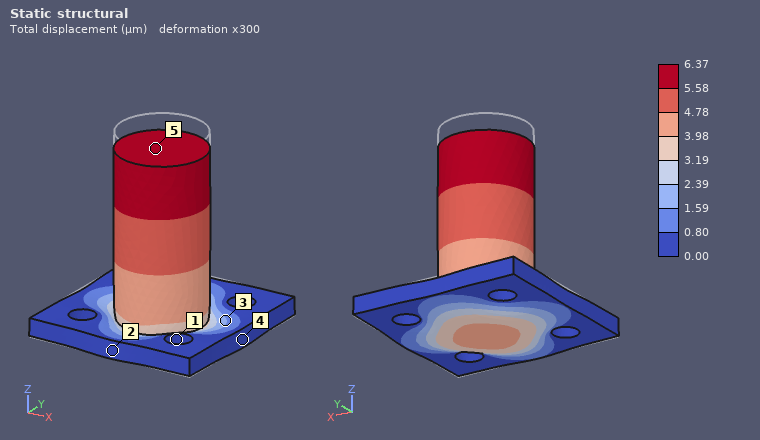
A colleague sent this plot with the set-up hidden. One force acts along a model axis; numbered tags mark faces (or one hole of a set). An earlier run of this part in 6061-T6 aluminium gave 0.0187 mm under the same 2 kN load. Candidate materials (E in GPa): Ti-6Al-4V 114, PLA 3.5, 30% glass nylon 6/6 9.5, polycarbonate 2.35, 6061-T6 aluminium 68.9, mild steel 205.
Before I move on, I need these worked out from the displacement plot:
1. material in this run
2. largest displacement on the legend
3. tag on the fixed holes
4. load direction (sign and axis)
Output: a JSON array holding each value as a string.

["mild steel", "6.37 µm", "1", "-Z"]
